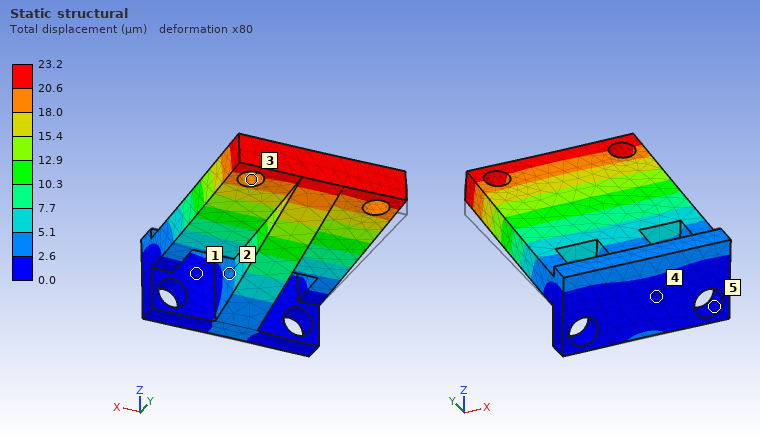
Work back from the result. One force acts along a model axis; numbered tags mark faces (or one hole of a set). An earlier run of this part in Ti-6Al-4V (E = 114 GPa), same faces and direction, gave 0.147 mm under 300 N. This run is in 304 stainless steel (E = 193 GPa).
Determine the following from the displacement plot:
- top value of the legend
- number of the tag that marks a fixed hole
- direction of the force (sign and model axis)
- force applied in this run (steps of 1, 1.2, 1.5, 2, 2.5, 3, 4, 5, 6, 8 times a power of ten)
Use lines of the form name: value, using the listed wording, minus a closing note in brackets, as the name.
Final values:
top value of the legend: 23.2 µm
number of the tag that marks a fixed hole: 5
direction of the force: +Z
force applied in this run: 80 N
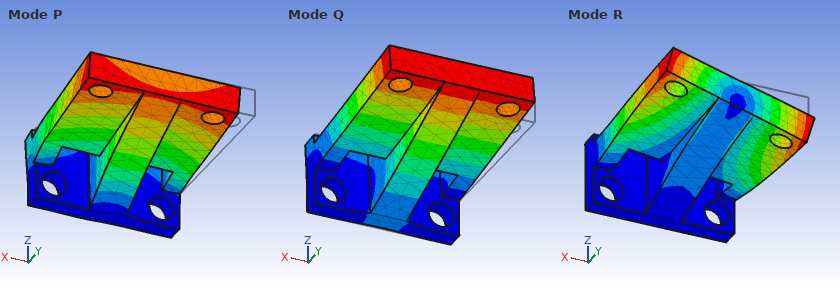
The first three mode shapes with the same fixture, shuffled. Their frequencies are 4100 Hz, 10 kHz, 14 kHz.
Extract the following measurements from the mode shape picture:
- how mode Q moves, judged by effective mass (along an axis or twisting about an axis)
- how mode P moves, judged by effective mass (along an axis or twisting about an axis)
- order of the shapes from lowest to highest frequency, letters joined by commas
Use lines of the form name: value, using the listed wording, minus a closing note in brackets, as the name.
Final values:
how mode Q moves, judged by effective mass: along Z
how mode P moves, judged by effective mass: along X
order of the shapes from lowest to highest frequency, letters joined by commas: Q, P, R
